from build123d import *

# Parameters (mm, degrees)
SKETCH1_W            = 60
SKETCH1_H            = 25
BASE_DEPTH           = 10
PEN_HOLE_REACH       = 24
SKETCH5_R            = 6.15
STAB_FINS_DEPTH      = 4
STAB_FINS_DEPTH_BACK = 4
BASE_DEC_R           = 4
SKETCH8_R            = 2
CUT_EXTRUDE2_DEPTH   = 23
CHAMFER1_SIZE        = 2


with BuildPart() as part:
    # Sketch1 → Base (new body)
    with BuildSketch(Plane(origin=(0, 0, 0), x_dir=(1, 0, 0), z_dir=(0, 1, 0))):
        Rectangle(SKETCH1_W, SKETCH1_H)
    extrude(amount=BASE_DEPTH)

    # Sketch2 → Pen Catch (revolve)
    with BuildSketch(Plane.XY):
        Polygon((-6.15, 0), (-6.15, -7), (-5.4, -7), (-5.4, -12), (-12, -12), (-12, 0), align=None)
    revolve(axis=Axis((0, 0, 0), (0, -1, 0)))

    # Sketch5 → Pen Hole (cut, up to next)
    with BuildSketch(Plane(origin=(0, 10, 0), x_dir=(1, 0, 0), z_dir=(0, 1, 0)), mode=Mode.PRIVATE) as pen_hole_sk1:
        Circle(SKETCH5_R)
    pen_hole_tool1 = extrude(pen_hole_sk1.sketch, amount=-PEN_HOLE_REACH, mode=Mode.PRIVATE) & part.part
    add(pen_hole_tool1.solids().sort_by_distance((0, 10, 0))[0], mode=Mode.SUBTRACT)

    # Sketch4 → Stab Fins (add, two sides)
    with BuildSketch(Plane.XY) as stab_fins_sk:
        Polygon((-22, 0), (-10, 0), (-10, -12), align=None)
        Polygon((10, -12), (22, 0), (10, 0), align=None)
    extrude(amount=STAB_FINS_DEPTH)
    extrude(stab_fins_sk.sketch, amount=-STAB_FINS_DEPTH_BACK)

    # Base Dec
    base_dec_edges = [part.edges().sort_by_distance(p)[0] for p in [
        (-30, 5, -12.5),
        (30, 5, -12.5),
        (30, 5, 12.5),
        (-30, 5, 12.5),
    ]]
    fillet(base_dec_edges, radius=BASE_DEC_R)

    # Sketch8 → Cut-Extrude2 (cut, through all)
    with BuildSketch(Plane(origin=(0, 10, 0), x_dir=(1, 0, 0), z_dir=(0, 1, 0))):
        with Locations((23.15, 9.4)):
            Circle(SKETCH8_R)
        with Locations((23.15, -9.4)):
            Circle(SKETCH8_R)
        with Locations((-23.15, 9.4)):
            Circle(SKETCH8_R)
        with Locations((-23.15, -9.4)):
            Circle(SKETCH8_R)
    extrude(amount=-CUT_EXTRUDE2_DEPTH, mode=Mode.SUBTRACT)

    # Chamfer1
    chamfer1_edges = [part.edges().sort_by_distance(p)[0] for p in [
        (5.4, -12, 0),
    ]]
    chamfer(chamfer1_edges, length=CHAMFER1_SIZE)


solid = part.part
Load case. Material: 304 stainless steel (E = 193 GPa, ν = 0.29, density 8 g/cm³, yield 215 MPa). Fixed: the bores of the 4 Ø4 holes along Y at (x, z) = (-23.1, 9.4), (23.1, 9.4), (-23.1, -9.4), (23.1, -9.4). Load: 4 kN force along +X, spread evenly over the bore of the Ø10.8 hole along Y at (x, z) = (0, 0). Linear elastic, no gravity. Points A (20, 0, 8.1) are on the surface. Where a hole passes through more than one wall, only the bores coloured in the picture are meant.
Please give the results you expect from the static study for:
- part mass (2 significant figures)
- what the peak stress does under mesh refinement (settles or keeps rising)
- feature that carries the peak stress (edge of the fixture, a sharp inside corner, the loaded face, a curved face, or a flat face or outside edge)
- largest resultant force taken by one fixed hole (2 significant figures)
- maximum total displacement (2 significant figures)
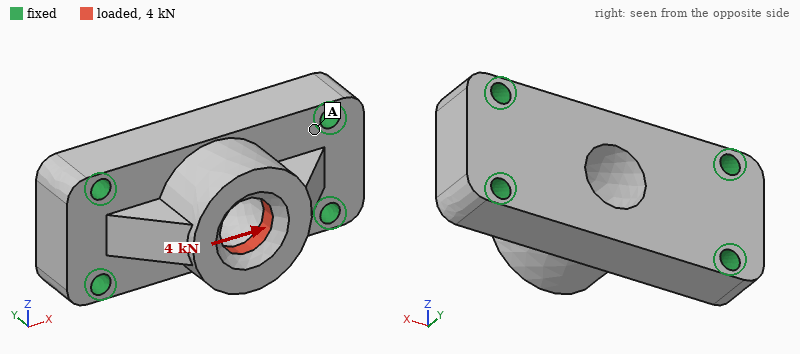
140 g
keeps rising
a sharp inside corner
1.2 kN
3.6 µm
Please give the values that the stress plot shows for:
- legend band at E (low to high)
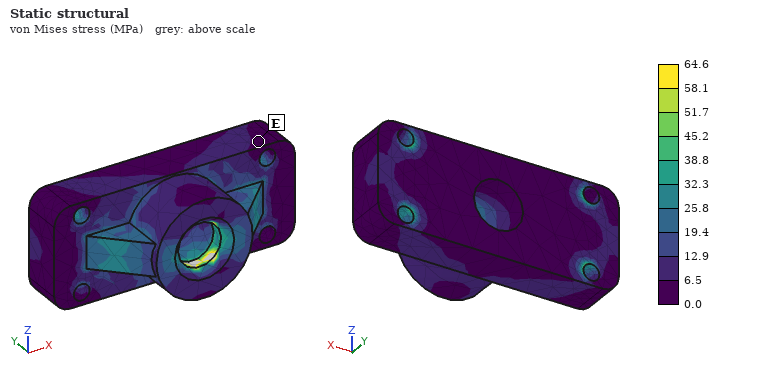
0.0 to 6.5 MPa
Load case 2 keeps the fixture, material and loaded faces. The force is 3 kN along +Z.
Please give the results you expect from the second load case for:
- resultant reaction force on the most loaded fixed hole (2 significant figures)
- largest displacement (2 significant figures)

1.5 kN
10 µm
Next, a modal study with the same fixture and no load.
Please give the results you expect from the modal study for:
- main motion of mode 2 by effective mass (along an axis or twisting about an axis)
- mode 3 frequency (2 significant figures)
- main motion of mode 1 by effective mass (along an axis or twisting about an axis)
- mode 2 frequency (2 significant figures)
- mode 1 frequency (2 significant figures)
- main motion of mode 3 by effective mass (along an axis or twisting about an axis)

along Y
28 kHz
along Z
18 kHz
16 kHz
along Z
